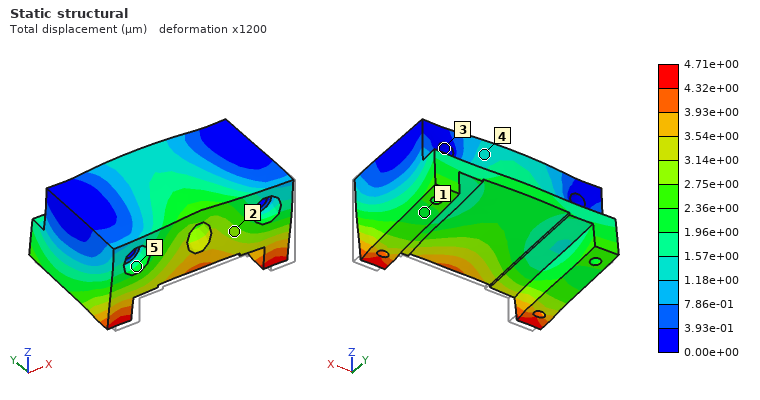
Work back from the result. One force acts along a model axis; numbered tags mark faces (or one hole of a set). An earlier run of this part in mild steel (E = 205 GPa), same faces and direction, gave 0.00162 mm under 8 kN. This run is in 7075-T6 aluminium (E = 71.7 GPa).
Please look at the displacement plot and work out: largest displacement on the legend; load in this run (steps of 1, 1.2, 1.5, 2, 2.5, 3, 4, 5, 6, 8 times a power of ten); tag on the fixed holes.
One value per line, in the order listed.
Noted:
4.71e+00 µm
8 kN
3
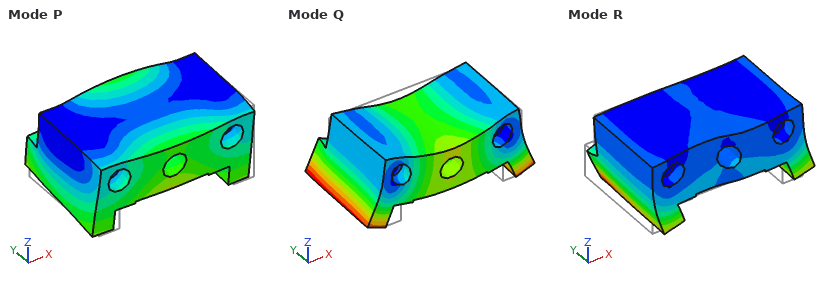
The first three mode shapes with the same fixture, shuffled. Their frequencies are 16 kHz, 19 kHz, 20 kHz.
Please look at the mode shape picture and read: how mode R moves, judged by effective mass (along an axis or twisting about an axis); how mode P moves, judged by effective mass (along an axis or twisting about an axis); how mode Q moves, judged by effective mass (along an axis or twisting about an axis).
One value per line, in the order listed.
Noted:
along X
along Y
along Z
